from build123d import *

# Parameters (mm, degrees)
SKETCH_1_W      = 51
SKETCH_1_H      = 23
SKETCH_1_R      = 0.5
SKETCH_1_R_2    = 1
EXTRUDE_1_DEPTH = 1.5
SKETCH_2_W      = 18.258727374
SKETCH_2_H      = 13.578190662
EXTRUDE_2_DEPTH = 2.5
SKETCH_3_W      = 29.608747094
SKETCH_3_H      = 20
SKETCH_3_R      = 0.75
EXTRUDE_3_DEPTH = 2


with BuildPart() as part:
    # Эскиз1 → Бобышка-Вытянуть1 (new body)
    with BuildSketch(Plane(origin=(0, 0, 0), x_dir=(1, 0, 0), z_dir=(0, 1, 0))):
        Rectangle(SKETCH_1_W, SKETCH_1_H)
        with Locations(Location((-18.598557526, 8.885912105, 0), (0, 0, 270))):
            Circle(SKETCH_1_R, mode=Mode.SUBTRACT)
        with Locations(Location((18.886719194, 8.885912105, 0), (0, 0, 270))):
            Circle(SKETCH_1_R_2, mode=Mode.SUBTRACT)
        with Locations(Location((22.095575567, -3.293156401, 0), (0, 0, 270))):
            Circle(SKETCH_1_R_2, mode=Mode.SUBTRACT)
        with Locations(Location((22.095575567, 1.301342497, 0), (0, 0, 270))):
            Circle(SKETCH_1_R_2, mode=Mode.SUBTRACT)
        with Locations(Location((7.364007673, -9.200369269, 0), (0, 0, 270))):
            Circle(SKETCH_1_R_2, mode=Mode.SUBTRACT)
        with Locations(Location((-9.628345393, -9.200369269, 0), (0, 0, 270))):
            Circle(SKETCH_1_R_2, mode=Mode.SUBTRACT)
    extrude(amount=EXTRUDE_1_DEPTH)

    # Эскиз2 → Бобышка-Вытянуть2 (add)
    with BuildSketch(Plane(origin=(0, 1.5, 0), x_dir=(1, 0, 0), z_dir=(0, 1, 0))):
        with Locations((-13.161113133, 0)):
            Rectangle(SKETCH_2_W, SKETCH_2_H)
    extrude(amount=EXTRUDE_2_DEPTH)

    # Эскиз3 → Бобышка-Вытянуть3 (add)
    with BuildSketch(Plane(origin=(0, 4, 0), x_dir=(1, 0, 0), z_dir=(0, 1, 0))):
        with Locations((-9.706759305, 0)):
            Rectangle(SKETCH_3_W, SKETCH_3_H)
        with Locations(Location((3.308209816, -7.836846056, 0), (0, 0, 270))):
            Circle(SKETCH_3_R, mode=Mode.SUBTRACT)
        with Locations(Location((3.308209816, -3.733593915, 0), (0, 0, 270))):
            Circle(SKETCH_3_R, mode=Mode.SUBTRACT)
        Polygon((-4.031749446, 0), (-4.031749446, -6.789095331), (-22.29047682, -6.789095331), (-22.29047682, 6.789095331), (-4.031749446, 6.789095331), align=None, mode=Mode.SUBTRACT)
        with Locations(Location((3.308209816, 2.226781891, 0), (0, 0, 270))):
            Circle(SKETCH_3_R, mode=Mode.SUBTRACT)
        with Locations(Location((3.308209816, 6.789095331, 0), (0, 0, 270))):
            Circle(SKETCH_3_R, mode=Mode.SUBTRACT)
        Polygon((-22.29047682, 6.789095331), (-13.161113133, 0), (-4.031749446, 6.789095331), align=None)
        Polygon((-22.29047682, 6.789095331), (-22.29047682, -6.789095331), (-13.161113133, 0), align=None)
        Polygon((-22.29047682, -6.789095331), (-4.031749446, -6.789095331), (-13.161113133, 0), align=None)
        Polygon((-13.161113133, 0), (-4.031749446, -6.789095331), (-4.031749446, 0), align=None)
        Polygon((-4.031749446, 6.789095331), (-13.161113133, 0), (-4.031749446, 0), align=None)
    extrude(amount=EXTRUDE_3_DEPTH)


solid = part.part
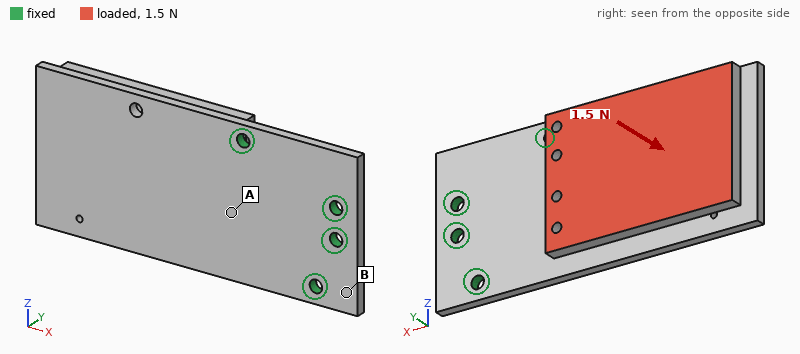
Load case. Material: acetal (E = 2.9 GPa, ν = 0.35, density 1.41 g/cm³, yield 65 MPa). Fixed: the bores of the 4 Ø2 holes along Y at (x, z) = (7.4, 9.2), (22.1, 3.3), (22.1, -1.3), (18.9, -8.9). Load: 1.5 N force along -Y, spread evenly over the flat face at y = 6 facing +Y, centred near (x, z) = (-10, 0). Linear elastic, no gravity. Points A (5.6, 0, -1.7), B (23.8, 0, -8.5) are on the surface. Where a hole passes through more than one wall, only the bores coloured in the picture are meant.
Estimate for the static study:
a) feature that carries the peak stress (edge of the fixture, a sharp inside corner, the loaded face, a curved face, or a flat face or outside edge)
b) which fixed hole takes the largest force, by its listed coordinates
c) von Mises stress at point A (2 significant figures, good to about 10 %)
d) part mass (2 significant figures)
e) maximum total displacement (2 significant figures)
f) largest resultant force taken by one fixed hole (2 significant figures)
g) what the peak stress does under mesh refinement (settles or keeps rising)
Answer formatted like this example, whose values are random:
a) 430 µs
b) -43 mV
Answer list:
a) edge of the fixture
b) (7.4, 9.2)
c) 1.9 MPa
d) 5.0 g
e) 0.51 mm
f) 2.0 N
g) keeps rising
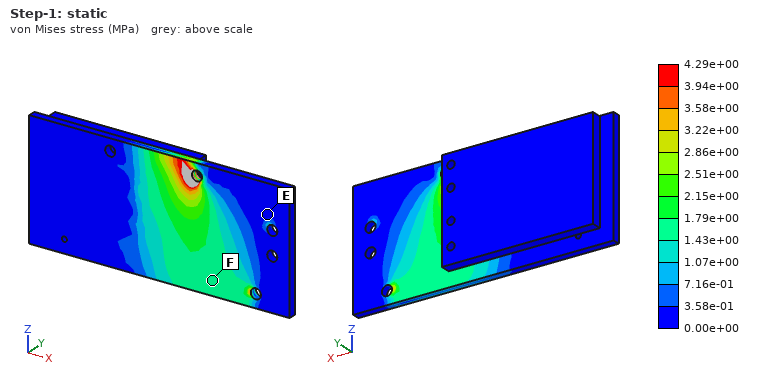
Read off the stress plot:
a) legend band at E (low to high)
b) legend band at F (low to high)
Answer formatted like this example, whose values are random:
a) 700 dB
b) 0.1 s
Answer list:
a) 0.00e+00 to 3.58e-01 MPa
b) 1.43e+00 to 1.79e+00 MPa
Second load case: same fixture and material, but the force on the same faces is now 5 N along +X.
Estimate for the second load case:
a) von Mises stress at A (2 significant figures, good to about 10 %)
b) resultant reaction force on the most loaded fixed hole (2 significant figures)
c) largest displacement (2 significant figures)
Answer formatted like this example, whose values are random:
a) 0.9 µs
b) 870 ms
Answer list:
a) 2.1 MPa
b) 2.0 N
c) 0.60 mm
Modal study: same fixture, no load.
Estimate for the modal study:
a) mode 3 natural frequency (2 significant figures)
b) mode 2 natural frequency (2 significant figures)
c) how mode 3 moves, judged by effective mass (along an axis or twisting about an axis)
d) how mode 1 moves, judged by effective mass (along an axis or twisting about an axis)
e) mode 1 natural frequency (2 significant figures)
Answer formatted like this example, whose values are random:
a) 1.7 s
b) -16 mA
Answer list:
a) 1300 Hz
b) 670 Hz
c) along Y
d) along Y
e) 170 Hz
